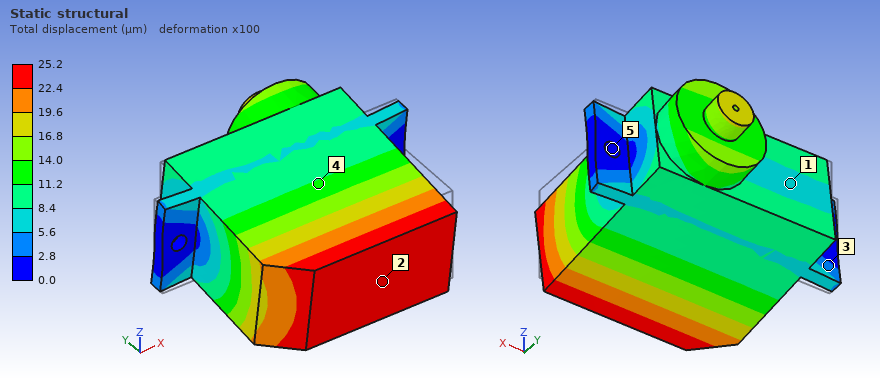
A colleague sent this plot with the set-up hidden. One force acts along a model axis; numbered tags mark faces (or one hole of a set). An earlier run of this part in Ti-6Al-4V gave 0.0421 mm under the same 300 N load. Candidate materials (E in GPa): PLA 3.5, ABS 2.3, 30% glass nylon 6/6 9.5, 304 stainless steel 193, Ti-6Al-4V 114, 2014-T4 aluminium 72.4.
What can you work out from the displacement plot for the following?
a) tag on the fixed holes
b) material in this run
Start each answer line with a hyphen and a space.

- 5
- 304 stainless steel
